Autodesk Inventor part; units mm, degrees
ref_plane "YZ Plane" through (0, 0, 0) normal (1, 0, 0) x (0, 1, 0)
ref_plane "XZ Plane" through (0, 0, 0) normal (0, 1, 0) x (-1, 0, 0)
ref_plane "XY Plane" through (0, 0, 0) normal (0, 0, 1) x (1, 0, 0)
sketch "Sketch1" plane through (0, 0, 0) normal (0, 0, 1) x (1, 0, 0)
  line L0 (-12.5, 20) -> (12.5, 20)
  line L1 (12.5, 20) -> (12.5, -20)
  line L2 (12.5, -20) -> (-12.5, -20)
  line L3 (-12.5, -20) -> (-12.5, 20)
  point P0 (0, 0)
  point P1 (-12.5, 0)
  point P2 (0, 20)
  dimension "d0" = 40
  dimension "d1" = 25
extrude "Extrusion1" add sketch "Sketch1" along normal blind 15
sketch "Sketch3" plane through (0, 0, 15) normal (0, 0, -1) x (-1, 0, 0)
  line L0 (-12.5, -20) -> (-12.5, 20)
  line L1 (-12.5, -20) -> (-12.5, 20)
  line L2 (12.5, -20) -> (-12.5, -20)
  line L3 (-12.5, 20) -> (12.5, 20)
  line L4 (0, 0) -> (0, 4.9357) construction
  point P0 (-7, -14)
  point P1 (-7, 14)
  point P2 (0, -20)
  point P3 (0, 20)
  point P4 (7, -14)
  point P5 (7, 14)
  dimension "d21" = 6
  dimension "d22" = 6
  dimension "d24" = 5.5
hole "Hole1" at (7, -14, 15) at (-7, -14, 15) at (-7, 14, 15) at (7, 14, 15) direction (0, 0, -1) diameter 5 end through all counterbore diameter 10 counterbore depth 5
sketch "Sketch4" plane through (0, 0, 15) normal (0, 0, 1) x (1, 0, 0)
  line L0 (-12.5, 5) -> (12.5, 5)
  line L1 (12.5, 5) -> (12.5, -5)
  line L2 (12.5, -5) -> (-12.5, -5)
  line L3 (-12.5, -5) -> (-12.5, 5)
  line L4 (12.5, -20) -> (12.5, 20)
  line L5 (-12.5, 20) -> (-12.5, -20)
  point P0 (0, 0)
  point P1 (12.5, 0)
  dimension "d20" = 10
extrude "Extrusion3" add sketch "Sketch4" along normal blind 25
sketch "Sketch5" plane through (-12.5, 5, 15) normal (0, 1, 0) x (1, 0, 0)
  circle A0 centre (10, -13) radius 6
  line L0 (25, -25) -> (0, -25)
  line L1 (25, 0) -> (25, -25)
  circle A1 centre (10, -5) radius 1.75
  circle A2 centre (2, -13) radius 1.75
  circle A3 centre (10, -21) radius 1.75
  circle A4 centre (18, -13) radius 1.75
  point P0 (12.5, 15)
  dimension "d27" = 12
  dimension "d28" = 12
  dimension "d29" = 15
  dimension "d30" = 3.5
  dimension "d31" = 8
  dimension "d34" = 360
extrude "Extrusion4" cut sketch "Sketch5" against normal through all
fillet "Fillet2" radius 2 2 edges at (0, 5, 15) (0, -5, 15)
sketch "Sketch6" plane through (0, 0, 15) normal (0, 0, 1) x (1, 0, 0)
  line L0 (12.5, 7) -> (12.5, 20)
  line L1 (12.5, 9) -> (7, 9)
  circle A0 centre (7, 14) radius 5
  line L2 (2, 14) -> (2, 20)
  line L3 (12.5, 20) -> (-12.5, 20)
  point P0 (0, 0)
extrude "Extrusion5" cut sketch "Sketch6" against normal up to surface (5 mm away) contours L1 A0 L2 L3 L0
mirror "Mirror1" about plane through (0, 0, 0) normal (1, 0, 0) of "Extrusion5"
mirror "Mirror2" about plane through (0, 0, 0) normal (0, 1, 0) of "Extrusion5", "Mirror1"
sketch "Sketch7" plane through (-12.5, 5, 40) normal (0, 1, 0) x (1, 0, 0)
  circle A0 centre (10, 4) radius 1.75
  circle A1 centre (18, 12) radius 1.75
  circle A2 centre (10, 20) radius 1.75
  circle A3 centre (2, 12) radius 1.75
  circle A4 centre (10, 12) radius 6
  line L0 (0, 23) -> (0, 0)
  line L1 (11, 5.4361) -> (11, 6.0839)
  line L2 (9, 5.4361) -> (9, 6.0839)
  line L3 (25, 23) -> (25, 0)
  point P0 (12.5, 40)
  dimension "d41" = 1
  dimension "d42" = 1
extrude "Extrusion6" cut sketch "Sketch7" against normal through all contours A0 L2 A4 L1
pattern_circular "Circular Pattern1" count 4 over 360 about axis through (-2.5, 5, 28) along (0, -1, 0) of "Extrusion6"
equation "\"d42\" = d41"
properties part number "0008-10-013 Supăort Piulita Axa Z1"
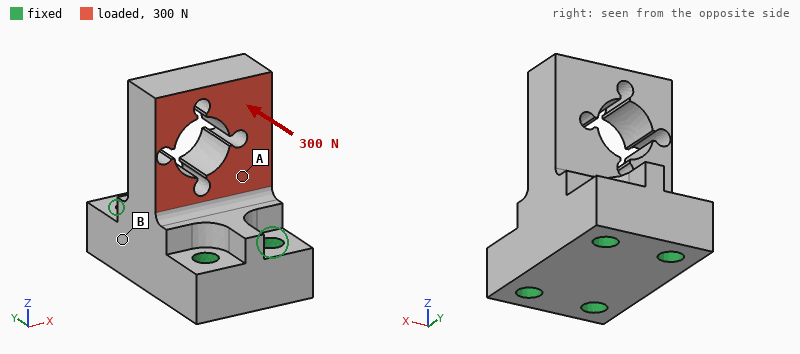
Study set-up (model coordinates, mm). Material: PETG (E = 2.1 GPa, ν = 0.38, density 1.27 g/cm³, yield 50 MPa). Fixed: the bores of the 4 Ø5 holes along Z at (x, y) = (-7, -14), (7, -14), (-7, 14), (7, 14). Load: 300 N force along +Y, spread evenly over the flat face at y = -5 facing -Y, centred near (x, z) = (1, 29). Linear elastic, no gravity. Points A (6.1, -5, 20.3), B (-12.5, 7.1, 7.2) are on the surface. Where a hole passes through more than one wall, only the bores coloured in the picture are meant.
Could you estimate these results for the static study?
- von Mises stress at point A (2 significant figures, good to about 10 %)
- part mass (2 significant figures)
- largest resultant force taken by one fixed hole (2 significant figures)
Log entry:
10 MPa
21 g
170 N
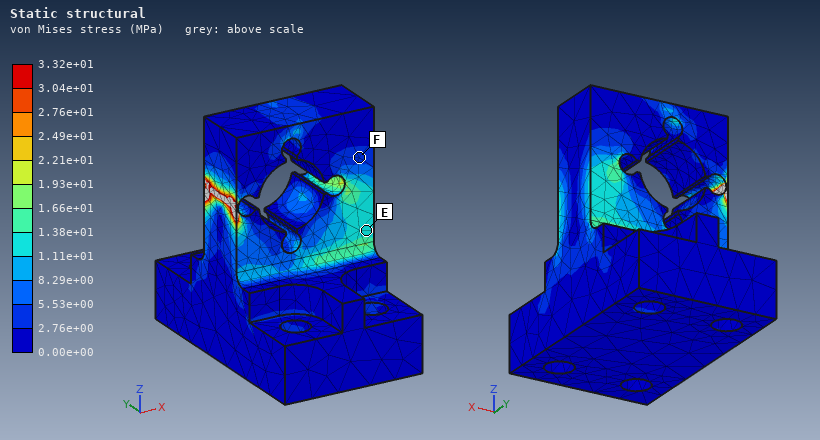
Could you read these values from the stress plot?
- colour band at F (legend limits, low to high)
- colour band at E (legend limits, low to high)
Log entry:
2.76e+00 to 5.53e+00 MPa
1.11e+01 to 1.38e+01 MPa
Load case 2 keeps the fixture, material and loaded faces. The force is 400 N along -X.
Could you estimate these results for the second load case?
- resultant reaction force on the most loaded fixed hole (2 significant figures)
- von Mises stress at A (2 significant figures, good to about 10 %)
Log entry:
300 N
8.5 MPa
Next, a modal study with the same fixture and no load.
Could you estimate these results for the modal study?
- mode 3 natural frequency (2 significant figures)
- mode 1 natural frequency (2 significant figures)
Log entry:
3800 Hz
1900 Hz
